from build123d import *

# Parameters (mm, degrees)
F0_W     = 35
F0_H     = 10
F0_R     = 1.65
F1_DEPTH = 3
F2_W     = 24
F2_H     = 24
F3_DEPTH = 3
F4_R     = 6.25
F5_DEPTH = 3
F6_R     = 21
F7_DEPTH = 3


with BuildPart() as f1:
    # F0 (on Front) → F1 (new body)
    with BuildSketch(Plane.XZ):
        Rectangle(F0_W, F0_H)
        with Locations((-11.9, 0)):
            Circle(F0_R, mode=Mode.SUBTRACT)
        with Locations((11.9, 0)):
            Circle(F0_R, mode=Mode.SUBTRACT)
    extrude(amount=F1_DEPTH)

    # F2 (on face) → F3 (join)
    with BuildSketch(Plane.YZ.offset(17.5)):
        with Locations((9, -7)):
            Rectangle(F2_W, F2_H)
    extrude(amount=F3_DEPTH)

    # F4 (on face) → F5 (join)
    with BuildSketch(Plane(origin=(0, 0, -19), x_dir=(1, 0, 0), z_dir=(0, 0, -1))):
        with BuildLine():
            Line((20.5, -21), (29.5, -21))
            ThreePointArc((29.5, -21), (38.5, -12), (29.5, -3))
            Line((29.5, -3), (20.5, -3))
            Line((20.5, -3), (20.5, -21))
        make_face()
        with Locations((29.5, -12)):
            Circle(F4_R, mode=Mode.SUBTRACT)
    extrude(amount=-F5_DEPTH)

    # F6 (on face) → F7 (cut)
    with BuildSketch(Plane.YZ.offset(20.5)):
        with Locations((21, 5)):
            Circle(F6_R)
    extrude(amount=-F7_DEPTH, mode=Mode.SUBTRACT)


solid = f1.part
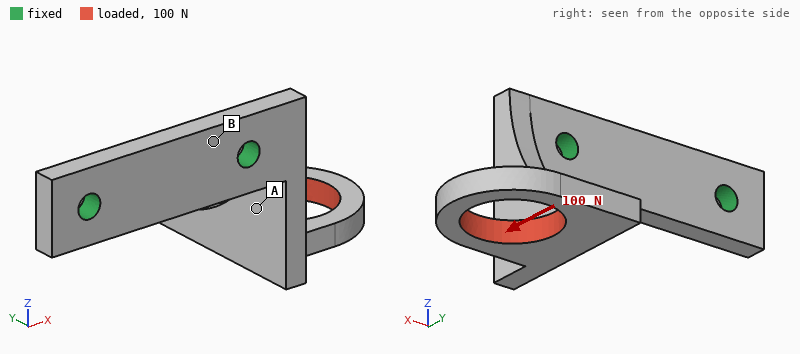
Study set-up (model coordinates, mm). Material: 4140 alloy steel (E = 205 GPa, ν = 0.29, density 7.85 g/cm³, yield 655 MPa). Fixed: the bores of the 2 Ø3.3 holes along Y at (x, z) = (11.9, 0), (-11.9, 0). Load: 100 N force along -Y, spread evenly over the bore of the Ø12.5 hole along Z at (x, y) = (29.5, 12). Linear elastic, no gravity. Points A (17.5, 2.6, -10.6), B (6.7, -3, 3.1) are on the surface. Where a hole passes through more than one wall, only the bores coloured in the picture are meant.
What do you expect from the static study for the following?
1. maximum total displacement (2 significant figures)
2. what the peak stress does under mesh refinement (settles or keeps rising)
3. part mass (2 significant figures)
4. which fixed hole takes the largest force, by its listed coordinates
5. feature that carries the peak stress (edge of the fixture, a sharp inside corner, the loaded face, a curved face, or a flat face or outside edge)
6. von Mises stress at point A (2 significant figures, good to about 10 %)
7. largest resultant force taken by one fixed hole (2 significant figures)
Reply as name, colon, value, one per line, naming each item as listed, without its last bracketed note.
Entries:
maximum total displacement: 0.22 mm
what the peak stress does under mesh refinement: keeps rising
part mass: 17 g
which fixed hole takes the largest force, by its listed coordinates: (11.9, 0)
feature that carries the peak stress: edge of the fixture
von Mises stress at point A: 72 MPa
largest resultant force taken by one fixed hole: 100 N
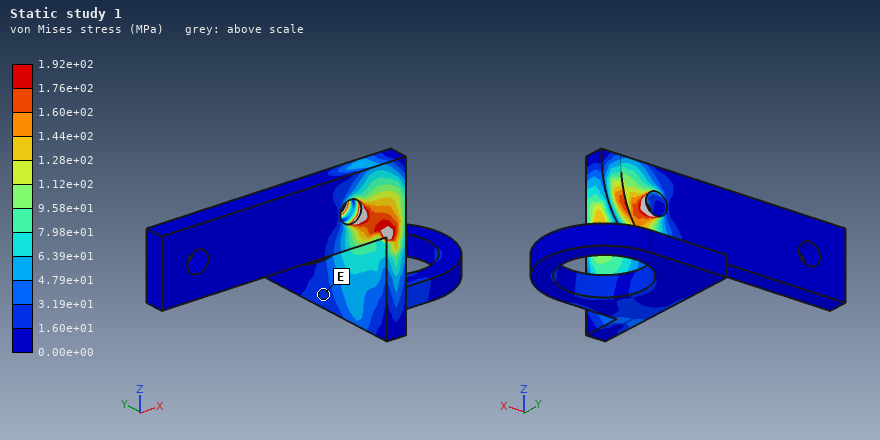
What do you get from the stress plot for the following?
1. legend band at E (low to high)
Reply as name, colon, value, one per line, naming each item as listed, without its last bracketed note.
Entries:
legend band at E: 1.60e+01 to 3.19e+01 MPa
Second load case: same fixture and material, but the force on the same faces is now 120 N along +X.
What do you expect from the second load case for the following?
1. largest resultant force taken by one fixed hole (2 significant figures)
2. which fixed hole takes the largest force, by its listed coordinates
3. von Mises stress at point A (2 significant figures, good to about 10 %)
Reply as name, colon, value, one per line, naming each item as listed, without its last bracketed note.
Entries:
largest resultant force taken by one fixed hole: 120 N
which fixed hole takes the largest force, by its listed coordinates: (11.9, 0)
von Mises stress at point A: 110 MPa
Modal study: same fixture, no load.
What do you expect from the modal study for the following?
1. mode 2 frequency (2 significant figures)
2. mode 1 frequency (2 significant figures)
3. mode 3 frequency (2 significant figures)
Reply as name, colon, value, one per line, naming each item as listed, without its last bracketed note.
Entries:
mode 2 frequency: 2000 Hz
mode 1 frequency: 1500 Hz
mode 3 frequency: 4100 Hz
